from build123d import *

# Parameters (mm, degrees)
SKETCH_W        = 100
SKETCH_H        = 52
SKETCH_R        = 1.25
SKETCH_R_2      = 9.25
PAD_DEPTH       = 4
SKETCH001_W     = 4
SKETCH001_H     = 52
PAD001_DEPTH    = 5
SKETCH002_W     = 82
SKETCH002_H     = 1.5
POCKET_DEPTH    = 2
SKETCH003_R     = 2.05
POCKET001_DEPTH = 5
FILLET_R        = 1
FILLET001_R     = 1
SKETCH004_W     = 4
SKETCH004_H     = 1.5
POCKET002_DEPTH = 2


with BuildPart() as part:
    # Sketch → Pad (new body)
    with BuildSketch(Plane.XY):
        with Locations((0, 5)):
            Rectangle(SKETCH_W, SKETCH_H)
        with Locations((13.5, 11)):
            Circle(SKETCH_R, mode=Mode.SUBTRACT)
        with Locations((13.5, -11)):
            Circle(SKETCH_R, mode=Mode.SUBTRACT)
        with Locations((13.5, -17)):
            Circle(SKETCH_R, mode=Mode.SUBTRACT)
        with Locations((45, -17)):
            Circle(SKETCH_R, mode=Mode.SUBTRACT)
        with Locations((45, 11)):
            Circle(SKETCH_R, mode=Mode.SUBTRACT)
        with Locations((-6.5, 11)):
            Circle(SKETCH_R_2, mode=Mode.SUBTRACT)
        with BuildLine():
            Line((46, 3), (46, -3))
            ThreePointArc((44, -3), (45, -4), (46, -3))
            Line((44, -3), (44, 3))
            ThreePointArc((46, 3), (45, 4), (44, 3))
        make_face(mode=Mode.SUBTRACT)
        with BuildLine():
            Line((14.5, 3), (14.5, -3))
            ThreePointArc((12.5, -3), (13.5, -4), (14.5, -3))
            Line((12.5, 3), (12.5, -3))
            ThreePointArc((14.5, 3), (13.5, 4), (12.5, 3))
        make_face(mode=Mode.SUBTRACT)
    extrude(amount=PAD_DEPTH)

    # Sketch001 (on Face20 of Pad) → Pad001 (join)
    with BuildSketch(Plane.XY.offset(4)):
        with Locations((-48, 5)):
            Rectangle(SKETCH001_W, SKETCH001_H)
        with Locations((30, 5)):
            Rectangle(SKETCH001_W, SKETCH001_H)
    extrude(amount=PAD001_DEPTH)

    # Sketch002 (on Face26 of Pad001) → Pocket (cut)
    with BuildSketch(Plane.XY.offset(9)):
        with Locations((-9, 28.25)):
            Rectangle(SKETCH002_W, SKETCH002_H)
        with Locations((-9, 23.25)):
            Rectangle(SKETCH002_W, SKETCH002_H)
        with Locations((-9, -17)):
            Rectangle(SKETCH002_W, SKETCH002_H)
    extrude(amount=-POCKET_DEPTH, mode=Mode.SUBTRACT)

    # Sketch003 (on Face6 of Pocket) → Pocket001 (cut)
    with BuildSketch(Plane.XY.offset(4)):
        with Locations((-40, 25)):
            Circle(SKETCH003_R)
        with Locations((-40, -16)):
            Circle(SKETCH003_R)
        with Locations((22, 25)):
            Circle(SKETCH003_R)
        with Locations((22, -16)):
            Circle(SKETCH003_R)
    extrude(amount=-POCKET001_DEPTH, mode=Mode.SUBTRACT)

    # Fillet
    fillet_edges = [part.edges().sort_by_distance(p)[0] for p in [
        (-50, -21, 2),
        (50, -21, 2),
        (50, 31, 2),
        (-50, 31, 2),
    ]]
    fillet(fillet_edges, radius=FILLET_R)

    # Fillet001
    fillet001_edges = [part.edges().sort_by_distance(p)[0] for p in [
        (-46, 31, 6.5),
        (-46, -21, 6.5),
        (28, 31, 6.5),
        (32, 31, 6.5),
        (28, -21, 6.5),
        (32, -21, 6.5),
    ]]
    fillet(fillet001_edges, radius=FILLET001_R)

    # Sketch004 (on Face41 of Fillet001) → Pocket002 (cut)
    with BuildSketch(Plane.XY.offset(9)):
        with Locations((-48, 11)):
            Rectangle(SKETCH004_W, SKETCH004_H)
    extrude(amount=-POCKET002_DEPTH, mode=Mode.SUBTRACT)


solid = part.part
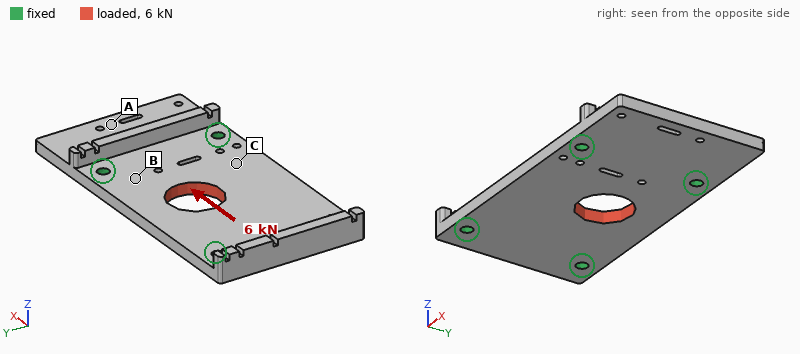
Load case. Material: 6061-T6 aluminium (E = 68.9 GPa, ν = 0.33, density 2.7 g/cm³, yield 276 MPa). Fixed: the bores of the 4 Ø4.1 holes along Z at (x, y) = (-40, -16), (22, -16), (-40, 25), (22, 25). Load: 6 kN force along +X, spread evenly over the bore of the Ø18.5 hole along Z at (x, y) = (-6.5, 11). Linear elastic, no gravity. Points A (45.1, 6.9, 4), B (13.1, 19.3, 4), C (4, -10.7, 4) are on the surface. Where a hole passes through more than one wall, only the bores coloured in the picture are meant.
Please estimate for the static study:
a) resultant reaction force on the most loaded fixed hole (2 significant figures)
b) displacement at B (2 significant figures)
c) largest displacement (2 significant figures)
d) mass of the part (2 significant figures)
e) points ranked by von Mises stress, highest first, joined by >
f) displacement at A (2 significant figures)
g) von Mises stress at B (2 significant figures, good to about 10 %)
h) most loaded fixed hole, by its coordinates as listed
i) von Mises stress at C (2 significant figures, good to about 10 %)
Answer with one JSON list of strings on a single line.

["2.0 kN", "5.0 µm", "11 µm", "57 g", "B > C > A", "3.5 µm", "27 MPa", "(22, 25)", "11 MPa"]
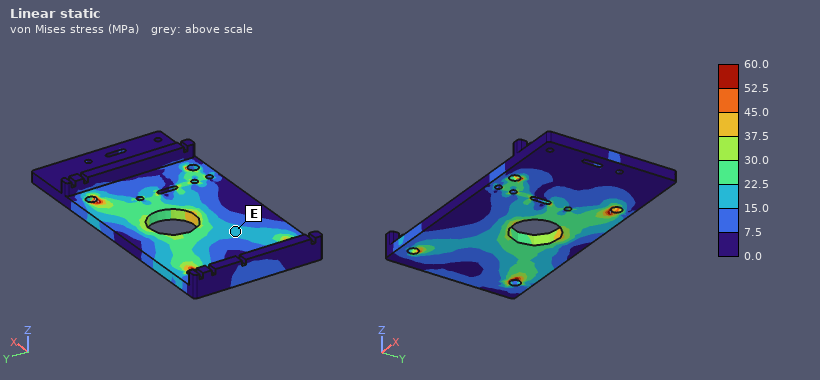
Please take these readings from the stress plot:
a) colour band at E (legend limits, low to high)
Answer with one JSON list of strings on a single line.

["15.0 to 22.5 MPa"]
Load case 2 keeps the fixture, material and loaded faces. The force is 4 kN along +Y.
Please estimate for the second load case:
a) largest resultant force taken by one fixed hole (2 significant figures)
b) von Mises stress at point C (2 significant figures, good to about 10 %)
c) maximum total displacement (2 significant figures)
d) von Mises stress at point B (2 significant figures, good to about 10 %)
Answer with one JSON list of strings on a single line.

["1.3 kN", "12 MPa", "19 µm", "24 MPa"]
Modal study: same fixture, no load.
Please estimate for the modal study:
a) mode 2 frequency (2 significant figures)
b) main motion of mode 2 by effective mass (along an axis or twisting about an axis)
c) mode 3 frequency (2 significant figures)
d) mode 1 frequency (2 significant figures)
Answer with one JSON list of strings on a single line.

["5000 Hz", "along Z", "6800 Hz", "3800 Hz"]
